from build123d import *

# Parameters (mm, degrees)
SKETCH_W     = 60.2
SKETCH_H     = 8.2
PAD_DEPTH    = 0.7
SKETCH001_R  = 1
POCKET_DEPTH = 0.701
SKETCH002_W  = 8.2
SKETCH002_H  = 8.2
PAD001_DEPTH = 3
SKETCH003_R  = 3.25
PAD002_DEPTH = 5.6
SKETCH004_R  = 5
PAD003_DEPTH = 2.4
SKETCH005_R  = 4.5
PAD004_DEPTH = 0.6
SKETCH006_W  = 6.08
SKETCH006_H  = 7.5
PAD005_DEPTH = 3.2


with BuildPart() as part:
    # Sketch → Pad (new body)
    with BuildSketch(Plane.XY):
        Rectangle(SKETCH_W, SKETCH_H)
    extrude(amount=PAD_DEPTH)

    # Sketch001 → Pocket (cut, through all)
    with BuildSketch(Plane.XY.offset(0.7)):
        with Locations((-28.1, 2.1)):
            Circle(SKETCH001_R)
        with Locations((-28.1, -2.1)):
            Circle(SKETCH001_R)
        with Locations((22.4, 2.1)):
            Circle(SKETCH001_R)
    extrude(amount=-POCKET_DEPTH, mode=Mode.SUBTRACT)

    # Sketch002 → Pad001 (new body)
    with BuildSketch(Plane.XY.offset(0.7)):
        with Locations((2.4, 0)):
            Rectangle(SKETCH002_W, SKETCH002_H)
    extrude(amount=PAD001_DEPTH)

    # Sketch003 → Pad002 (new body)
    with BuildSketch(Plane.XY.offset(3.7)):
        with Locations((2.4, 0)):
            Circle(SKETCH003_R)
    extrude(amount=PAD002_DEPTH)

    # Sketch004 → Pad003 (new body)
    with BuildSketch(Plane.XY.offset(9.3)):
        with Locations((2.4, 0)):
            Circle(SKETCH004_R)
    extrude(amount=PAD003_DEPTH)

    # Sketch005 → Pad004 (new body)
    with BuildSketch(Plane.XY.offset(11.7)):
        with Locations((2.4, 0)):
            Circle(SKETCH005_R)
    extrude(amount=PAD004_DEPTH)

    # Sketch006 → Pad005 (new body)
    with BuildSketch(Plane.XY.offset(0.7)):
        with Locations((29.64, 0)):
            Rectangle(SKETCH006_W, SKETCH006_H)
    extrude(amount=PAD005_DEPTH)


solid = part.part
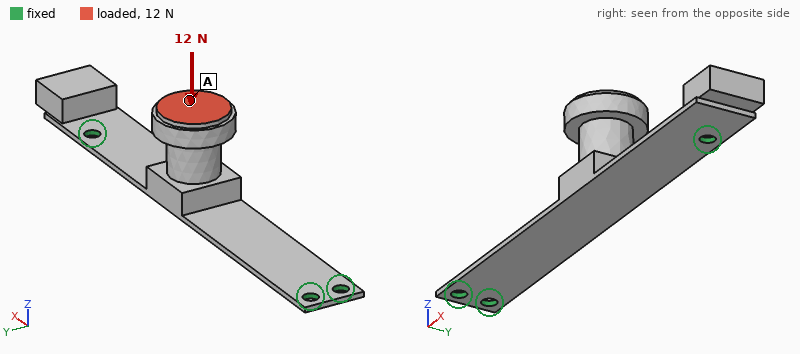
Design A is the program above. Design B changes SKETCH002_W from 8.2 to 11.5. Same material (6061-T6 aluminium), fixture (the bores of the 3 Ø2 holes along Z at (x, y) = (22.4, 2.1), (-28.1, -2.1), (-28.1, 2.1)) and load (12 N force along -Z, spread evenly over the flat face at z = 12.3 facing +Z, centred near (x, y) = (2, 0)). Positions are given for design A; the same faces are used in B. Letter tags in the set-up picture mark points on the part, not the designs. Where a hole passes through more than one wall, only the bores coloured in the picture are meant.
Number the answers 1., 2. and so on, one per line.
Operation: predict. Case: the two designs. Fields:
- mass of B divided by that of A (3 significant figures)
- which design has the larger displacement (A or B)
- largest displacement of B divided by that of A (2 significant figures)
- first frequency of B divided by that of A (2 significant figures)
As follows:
1. 1.07
2. A
3. 0.84
4. 1.0
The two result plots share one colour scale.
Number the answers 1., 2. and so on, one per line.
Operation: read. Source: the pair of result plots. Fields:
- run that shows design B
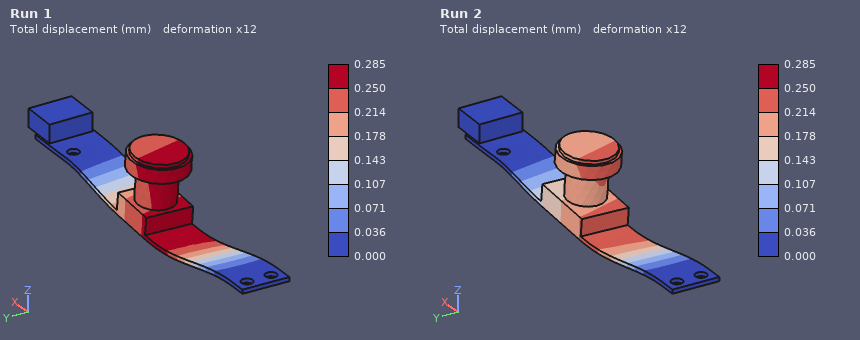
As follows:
1. Run 2
